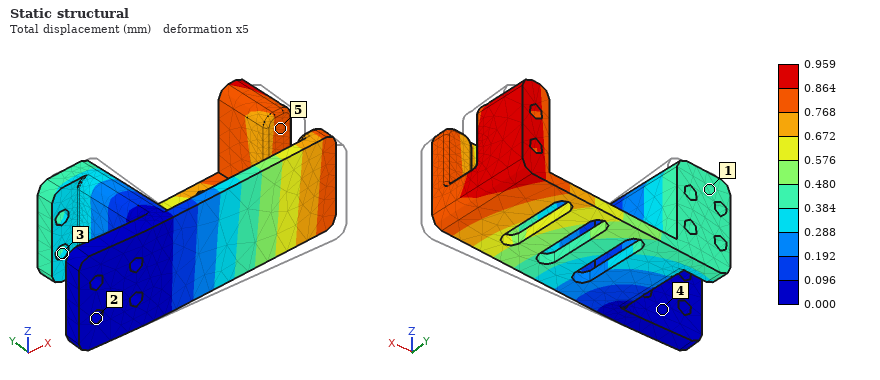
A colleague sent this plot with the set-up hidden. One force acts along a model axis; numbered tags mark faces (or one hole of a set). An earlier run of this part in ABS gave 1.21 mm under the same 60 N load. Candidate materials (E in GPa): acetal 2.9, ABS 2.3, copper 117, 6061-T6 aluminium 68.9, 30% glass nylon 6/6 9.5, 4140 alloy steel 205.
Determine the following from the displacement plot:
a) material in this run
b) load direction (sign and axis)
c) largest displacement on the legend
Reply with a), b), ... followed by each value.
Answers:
a) acetal
b) -X
c) 0.959 mm
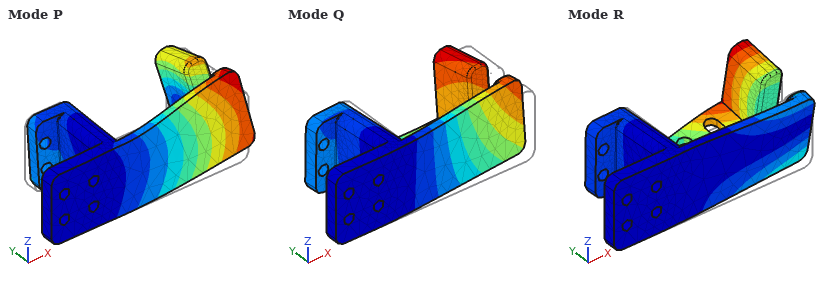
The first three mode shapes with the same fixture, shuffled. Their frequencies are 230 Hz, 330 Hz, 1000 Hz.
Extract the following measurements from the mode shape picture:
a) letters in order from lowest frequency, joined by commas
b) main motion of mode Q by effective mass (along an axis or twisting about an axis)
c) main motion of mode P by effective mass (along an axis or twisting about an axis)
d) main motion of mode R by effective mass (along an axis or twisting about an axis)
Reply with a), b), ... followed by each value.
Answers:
a) Q, R, P
b) along Y
c) along Z
d) along Z
